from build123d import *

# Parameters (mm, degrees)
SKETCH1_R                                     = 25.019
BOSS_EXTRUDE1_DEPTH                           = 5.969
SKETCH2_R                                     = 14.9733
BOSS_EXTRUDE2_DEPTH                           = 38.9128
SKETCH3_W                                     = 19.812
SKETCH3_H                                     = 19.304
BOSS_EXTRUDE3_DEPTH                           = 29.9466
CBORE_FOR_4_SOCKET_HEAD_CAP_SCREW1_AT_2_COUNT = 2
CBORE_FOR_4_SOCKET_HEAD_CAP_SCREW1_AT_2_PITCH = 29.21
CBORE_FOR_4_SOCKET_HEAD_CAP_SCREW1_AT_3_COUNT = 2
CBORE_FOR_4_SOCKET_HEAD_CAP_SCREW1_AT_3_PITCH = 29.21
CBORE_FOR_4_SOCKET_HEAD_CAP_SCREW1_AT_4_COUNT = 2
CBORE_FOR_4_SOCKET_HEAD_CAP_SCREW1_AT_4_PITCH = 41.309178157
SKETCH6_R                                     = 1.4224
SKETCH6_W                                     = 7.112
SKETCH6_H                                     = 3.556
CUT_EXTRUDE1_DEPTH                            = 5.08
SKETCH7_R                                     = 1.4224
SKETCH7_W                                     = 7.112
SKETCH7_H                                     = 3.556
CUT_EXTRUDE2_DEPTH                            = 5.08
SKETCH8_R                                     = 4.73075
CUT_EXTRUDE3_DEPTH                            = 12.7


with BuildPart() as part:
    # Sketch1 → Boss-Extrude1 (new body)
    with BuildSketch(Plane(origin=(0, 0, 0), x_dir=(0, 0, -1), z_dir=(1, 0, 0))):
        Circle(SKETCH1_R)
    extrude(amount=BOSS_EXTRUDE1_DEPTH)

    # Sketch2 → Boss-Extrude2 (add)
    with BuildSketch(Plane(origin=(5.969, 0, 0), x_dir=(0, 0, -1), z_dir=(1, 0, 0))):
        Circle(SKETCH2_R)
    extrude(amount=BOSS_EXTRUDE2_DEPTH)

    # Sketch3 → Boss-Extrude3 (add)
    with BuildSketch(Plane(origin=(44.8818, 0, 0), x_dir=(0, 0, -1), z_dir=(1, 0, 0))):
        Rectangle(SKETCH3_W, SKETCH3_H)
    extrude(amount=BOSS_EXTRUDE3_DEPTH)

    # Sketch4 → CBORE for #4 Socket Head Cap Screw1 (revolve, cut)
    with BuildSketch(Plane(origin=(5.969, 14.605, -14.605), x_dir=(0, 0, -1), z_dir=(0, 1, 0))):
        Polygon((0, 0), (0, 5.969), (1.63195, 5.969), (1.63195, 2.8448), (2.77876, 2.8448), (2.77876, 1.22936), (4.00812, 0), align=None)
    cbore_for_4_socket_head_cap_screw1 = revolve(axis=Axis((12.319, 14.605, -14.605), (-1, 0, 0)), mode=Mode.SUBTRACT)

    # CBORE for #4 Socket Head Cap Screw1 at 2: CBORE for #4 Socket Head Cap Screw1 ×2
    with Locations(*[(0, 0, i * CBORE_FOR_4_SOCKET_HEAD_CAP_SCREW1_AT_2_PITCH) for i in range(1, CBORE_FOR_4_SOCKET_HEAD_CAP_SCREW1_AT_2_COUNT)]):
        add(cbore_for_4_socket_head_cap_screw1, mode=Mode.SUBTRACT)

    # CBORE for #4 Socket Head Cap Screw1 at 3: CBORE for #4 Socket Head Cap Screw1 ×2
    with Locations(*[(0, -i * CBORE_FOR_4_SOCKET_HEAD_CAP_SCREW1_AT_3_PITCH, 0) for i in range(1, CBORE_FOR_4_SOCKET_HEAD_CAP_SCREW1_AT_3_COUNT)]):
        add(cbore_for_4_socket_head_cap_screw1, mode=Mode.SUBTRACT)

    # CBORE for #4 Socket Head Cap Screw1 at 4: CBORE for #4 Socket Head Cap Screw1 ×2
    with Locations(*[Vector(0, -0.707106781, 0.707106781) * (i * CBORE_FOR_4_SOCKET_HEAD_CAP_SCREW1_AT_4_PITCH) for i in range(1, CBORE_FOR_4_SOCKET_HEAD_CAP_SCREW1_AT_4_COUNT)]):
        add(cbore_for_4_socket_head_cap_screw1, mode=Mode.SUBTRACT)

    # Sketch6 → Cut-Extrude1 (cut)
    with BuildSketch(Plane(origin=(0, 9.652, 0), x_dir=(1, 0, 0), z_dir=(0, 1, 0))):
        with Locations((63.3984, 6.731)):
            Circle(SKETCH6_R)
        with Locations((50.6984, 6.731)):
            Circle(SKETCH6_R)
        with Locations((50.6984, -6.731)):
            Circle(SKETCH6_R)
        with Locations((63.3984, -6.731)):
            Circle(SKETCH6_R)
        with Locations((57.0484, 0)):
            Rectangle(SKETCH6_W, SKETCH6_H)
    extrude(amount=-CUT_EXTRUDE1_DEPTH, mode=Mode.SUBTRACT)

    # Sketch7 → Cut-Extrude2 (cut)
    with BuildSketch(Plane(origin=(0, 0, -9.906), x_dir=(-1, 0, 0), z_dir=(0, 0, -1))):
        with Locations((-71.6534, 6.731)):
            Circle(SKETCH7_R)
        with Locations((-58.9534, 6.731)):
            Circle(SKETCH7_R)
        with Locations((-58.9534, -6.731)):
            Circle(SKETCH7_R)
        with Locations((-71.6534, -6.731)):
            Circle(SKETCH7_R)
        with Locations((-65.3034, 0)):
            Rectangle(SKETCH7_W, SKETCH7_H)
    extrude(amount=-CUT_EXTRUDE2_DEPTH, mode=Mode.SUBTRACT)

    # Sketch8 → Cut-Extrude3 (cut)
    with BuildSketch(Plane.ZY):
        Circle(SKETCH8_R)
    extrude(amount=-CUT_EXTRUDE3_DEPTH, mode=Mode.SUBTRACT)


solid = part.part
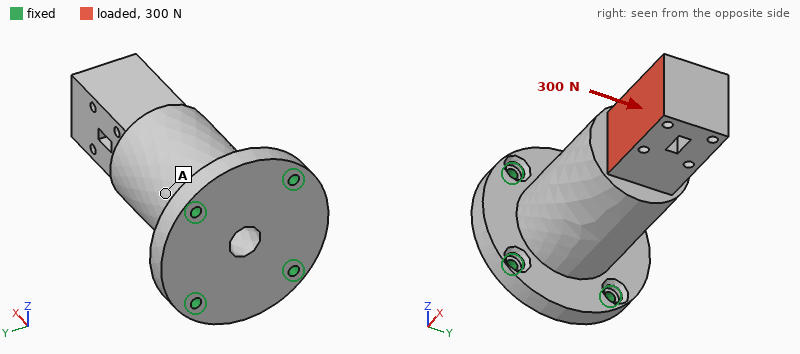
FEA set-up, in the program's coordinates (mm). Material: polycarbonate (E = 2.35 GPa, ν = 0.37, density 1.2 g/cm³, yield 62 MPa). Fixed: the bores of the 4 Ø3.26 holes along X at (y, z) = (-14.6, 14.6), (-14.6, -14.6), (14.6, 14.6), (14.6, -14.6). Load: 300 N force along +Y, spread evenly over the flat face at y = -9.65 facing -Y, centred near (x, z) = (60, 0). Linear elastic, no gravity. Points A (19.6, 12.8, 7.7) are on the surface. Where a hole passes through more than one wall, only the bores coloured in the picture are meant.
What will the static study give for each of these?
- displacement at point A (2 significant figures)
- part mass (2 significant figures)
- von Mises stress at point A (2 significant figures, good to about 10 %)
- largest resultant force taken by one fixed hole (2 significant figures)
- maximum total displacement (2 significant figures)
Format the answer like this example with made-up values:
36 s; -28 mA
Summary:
0.17 mm; 58 g; 3.9 MPa; 350 N; 0.78 mm
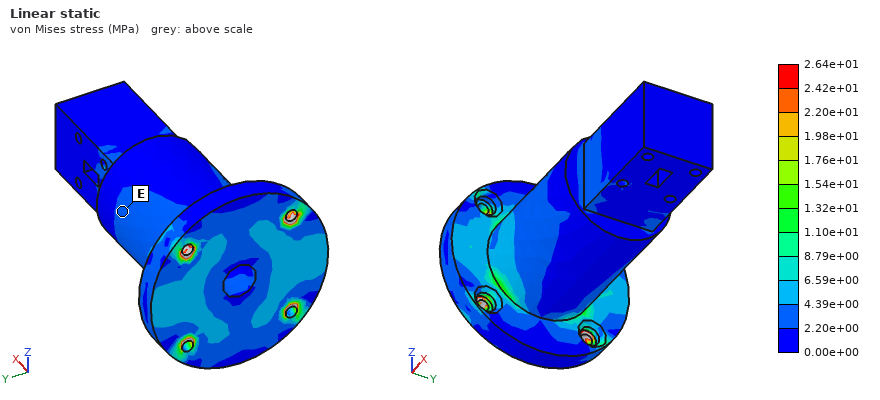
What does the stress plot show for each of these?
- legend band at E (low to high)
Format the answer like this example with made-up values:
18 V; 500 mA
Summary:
2.20e+00 to 4.39e+00 MPa
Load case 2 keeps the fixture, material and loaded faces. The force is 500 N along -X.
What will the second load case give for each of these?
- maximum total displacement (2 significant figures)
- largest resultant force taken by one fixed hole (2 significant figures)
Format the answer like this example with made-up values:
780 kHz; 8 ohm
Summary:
0.32 mm; 240 N
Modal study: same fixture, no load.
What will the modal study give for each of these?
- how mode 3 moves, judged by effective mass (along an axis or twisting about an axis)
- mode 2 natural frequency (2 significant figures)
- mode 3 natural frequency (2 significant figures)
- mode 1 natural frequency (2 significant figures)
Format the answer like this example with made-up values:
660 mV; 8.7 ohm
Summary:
along X; 840 Hz; 2500 Hz; 840 Hz
